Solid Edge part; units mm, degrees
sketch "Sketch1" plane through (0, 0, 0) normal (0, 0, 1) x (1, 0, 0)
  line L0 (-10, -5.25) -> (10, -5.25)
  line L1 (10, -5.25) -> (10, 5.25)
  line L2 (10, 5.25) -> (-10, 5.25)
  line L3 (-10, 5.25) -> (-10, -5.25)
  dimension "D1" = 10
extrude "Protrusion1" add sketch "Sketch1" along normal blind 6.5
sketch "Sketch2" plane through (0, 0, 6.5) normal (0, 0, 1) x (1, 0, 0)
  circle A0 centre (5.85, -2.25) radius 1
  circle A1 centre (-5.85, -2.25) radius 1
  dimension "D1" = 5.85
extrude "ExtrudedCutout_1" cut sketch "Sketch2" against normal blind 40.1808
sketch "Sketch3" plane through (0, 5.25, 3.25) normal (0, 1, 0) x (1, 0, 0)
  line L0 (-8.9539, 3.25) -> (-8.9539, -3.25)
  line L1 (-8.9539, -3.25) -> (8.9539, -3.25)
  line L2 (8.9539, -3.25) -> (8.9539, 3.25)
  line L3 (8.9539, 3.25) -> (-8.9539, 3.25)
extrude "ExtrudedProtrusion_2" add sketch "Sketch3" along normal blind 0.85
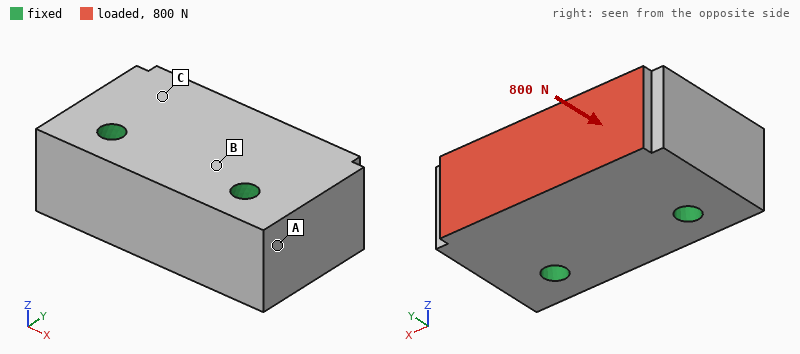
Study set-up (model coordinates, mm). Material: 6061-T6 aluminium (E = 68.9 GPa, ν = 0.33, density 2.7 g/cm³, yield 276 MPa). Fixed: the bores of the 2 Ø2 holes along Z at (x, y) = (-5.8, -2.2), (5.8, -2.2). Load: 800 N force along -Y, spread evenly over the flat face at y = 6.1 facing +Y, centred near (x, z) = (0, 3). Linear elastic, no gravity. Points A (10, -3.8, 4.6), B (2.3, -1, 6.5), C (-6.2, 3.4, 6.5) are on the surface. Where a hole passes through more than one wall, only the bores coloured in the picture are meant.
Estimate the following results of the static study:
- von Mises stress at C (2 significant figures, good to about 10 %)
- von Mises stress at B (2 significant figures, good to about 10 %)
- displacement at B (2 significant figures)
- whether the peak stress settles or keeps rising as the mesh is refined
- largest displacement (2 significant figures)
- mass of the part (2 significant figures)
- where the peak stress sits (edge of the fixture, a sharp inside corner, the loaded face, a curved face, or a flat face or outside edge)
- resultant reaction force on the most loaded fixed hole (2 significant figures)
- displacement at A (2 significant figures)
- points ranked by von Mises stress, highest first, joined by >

7.7 MPa
4.3 MPa
0.56 µm
keeps rising
1.1 µm
3.8 g
edge of the fixture
410 N
0.35 µm
C > B > A
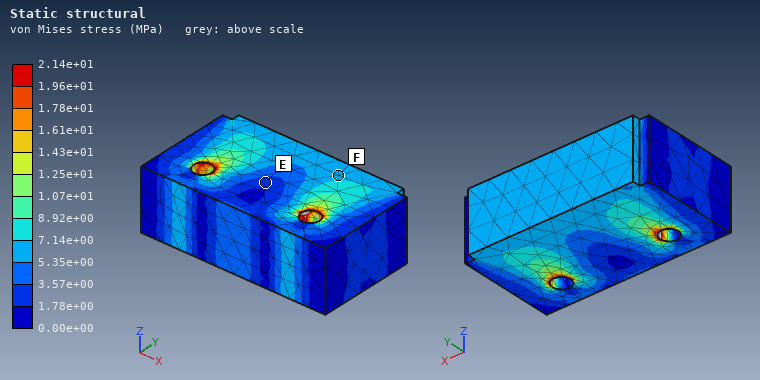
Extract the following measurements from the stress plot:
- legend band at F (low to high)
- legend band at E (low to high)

5.35e+00 to 7.14e+00 MPa
1.78e+00 to 3.57e+00 MPa
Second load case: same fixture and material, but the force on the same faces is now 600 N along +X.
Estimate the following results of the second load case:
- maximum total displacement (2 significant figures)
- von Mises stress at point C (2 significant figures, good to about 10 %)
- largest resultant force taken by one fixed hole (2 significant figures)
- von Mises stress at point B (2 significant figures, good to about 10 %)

3.3 µm
6.7 MPa
470 N
9.3 MPa
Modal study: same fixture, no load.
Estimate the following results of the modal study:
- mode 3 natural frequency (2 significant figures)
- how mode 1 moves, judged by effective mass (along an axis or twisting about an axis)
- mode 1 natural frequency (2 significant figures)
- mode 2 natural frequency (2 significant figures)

69 kHz
along Z
47 kHz
66 kHz
